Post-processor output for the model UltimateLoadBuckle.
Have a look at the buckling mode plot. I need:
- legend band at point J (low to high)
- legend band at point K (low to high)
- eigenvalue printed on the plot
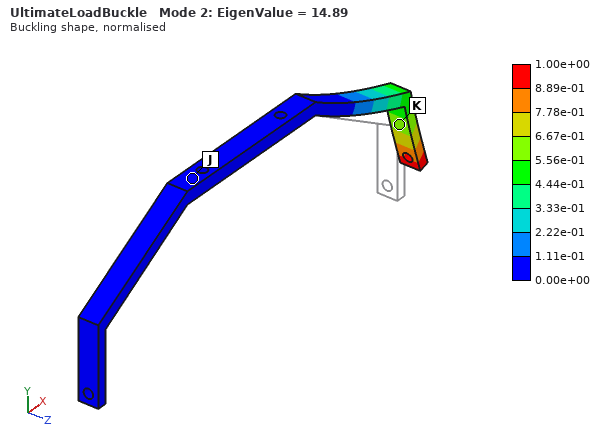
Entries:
0.00e+00 to 1.11e-01
5.56e-01 to 6.67e-01
14.89
